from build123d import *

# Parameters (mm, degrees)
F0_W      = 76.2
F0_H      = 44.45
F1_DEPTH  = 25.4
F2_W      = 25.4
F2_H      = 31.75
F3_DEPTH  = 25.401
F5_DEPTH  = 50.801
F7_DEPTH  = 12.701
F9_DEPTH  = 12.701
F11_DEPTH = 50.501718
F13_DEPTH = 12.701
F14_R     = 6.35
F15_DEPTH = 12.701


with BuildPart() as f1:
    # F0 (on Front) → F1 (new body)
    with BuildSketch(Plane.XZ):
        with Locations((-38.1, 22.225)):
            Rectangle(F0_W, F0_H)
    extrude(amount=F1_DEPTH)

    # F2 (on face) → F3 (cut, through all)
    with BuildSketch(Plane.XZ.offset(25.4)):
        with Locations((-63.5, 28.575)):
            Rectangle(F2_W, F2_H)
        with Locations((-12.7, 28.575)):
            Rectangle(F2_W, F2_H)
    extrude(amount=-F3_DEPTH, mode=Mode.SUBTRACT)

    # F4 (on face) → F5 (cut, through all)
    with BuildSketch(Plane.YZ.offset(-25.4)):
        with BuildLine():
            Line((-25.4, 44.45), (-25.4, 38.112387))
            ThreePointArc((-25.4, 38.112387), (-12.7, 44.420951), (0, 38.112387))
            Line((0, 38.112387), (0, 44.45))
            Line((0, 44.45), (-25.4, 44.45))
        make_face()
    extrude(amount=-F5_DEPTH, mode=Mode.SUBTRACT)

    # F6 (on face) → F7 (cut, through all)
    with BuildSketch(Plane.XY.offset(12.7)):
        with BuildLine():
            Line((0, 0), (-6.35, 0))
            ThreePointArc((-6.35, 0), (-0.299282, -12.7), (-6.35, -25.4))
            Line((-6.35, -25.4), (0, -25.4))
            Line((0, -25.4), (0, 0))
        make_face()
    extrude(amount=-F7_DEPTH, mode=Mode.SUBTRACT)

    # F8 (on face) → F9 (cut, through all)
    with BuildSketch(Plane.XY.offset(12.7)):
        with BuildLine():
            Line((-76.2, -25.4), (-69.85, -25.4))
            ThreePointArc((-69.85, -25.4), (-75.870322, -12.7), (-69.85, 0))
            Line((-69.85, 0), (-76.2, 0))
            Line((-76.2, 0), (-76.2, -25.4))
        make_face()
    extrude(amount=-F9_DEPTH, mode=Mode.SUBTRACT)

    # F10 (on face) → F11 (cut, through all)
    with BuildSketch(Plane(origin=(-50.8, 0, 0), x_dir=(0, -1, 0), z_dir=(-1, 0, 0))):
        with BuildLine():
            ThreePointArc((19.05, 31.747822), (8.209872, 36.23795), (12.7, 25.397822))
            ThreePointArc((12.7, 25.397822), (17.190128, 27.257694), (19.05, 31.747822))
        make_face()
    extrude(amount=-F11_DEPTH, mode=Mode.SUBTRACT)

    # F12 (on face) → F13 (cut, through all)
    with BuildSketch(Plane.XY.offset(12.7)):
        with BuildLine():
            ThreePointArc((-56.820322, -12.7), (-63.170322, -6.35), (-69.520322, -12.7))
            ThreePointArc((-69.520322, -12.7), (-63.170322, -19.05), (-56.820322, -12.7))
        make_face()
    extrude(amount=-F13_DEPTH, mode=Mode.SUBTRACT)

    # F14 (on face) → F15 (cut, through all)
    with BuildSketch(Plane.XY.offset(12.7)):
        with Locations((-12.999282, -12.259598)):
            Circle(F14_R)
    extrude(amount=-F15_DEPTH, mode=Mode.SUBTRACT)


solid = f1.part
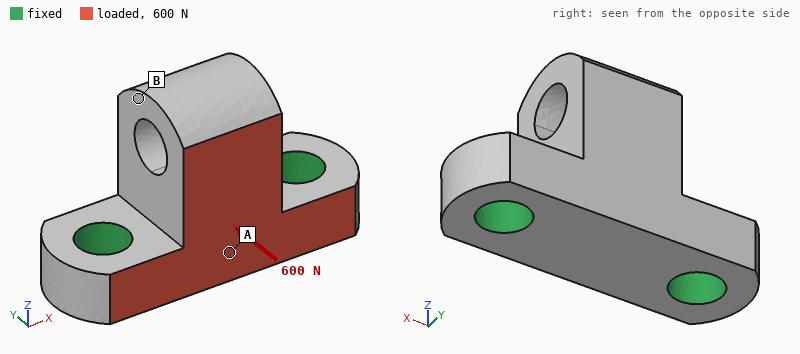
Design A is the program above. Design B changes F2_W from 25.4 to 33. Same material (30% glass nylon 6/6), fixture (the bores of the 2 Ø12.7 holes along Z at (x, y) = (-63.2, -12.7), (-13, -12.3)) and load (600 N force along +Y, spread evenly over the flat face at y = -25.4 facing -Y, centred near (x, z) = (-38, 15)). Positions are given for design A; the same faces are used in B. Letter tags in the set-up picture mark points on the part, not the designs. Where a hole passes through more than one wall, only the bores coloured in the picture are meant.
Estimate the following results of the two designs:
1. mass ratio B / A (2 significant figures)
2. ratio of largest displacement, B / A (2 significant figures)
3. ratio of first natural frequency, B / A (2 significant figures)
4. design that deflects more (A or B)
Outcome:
0.87
1.1
1.0
B
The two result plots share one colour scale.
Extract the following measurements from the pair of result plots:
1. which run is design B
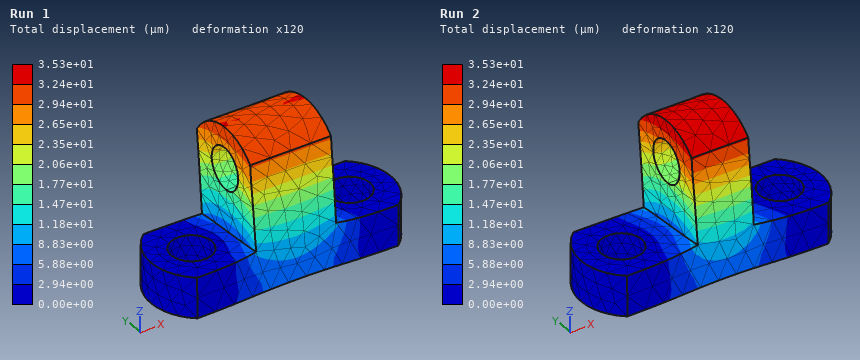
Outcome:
Run 2
